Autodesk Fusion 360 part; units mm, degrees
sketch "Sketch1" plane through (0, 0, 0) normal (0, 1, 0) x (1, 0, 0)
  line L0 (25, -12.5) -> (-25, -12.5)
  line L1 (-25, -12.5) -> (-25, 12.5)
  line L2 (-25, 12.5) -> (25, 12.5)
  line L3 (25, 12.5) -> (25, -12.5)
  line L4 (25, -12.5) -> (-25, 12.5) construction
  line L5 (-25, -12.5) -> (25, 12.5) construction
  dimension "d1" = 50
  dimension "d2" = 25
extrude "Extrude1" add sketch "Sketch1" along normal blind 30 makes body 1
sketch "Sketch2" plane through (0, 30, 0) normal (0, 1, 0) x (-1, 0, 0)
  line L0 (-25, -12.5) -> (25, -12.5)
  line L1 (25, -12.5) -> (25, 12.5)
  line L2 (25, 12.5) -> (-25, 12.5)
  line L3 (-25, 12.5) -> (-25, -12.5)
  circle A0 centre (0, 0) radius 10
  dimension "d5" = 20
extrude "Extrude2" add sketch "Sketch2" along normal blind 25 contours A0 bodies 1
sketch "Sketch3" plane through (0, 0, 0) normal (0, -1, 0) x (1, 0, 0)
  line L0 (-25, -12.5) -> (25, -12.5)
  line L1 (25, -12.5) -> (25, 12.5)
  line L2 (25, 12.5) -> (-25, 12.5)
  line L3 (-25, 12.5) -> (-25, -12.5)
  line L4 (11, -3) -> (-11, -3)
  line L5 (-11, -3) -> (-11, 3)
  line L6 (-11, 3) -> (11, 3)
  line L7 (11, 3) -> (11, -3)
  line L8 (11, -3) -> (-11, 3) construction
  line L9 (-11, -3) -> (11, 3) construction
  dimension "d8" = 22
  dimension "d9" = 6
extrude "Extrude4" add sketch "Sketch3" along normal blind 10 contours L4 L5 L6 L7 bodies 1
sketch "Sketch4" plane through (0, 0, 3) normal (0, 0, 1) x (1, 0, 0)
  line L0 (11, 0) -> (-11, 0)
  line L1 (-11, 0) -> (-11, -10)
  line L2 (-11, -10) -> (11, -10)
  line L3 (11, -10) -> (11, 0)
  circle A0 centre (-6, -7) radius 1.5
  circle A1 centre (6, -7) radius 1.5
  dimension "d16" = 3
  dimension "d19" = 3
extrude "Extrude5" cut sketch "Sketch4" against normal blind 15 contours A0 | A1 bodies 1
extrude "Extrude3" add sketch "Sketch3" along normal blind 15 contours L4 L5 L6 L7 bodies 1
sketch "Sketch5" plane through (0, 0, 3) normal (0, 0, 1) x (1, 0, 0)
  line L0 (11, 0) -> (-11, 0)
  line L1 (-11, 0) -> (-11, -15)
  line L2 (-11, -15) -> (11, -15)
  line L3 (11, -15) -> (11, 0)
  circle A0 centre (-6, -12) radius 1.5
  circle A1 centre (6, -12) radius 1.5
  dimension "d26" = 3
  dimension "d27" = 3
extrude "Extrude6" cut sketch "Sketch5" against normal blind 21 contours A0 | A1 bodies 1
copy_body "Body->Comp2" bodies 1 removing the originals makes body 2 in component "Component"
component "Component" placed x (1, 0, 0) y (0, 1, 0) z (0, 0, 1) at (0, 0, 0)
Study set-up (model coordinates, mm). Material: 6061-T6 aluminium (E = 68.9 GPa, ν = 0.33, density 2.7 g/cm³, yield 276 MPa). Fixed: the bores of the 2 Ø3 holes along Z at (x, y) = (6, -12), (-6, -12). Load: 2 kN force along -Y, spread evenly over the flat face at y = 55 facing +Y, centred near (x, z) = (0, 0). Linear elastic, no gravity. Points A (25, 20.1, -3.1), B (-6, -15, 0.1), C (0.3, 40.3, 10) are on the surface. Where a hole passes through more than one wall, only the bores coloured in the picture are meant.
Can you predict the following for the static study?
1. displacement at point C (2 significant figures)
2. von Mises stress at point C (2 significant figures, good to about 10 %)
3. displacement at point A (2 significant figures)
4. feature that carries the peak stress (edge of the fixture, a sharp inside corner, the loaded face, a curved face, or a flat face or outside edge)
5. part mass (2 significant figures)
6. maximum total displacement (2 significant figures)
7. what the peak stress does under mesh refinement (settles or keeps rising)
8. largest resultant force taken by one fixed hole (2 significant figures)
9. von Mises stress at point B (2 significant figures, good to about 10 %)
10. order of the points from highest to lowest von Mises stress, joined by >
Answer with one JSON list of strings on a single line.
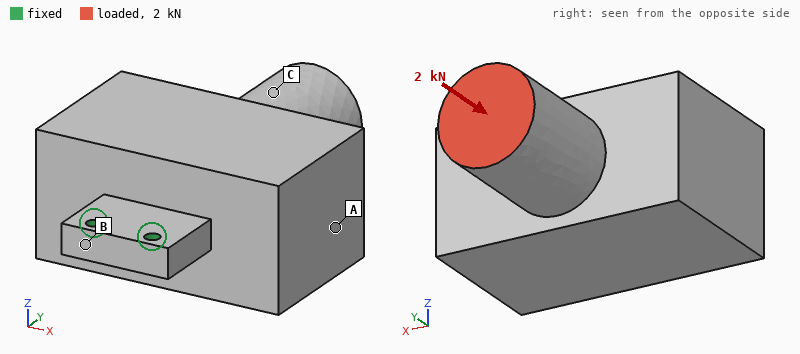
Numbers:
["5.9 µm", "6.2 MPa", "4.1 µm", "edge of the fixture", "130 g", "7.3 µm", "keeps rising", "1.0 kN", "12 MPa", "B > C > A"]
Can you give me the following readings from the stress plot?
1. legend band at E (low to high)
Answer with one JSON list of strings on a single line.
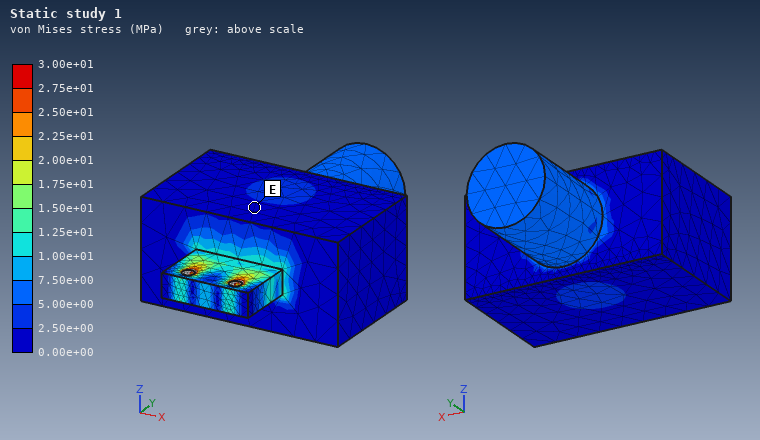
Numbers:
["0.00e+00 to 2.50e+00 MPa"]
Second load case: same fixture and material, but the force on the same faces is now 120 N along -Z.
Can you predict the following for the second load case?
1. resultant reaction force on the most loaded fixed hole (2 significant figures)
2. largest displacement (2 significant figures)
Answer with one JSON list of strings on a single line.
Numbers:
["60 N", "0.22 mm"]
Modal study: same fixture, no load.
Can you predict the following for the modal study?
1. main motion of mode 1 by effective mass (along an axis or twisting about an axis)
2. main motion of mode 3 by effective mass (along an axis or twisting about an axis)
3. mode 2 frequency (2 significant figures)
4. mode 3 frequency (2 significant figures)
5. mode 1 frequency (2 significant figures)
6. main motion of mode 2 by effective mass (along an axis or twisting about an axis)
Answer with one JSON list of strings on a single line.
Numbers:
["along Z", "twisting about Y", "2000 Hz", "2200 Hz", "690 Hz", "along X"]
